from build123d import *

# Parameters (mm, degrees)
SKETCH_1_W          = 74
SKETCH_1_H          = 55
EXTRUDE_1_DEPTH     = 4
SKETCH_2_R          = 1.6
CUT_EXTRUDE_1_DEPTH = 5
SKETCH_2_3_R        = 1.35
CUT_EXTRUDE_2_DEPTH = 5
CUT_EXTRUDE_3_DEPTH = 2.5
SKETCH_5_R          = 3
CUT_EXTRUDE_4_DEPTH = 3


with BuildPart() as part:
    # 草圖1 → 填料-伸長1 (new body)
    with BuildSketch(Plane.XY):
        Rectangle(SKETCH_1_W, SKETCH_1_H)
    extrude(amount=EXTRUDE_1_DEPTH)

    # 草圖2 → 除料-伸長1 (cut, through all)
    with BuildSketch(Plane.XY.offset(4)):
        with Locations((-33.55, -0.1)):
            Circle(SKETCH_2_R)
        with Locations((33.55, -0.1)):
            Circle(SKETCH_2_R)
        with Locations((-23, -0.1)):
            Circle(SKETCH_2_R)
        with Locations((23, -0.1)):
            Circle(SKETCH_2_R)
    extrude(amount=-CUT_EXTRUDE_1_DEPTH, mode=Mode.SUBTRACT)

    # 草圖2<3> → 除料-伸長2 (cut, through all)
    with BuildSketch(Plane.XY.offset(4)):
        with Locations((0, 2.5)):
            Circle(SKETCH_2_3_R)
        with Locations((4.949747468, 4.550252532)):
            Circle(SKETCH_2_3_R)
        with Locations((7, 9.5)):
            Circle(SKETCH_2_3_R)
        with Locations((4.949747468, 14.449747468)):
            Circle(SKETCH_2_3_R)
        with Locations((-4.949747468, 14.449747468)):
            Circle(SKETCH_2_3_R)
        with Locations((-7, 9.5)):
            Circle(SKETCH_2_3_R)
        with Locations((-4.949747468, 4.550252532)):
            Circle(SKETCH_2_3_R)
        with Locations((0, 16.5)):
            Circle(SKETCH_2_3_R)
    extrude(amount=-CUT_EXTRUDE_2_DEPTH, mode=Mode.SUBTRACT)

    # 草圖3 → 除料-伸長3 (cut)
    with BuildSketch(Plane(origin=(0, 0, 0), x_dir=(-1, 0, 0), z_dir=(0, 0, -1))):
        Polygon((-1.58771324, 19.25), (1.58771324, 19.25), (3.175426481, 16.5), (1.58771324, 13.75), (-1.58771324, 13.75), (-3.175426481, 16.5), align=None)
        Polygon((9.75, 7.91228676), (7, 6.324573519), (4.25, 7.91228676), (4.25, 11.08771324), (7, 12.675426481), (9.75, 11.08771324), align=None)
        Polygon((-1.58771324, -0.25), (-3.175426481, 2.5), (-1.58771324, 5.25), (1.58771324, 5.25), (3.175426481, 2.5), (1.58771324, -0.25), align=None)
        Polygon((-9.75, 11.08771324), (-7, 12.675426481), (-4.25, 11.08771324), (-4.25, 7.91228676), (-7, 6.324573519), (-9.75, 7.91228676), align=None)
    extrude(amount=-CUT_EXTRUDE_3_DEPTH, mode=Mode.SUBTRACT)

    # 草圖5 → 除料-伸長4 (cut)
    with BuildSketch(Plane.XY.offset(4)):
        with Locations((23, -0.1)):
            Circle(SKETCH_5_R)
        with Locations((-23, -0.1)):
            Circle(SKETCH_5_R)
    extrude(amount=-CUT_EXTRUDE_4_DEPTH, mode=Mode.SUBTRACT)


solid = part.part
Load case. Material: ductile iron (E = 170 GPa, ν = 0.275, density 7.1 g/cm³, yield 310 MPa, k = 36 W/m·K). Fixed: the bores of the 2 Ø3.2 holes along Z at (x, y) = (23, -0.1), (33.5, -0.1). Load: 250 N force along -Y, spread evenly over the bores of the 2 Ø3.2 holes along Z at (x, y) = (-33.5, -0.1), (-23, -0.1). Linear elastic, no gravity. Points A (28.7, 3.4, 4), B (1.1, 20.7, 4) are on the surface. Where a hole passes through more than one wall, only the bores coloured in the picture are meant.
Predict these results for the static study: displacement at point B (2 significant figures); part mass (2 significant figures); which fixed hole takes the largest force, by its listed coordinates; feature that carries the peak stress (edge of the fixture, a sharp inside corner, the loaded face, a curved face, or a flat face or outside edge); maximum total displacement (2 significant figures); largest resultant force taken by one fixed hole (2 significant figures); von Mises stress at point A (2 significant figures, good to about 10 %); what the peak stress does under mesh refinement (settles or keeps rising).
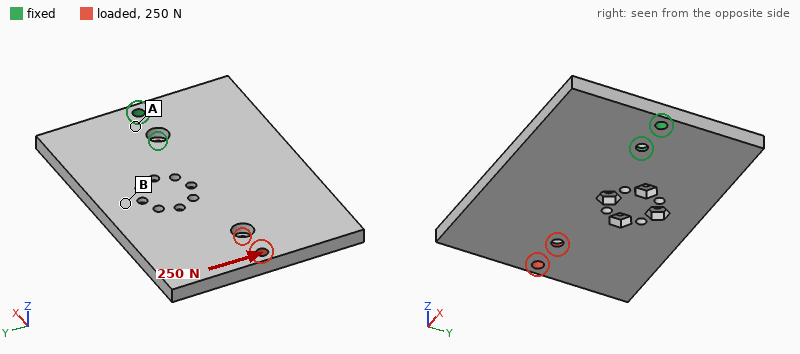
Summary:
20 µm
110 g
(23, -0.1)
edge of the fixture
37 µm
1.2 kN
15 MPa
keeps rising
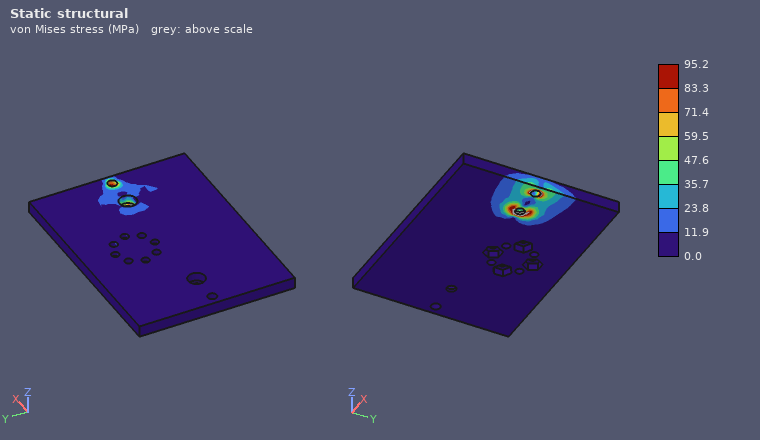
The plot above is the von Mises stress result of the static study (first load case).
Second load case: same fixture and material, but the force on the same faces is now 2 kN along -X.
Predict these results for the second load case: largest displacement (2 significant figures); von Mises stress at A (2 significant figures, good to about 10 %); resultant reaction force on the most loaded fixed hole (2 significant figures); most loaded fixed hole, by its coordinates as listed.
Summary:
18 µm
29 MPa
1.1 kN
(33.5, -0.1)
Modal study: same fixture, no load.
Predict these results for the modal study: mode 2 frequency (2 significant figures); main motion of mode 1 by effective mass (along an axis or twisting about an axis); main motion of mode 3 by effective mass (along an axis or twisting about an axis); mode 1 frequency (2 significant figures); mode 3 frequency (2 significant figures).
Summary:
1200 Hz
along Z
along Y
680 Hz
2400 Hz
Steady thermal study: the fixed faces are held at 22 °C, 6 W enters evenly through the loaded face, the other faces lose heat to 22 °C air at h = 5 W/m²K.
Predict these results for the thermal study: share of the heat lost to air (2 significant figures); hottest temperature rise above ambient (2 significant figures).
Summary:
22 %
67 K
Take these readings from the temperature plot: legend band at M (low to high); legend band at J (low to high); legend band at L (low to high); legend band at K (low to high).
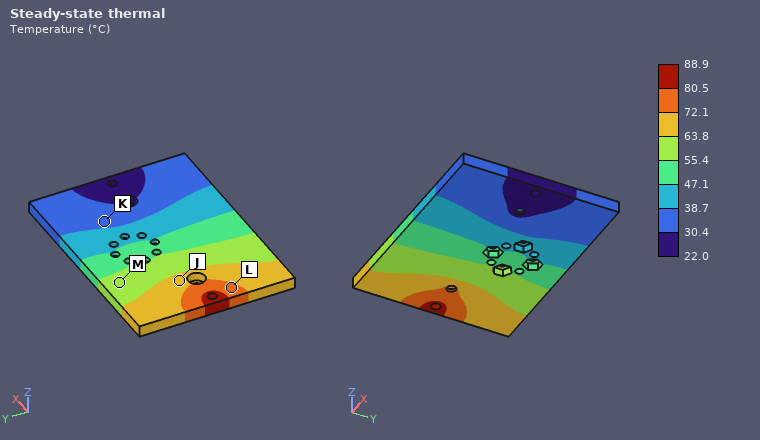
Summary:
55.4 to 63.8 °C
63.8 to 72.1 °C
72.1 to 80.5 °C
30.4 to 38.7 °C
